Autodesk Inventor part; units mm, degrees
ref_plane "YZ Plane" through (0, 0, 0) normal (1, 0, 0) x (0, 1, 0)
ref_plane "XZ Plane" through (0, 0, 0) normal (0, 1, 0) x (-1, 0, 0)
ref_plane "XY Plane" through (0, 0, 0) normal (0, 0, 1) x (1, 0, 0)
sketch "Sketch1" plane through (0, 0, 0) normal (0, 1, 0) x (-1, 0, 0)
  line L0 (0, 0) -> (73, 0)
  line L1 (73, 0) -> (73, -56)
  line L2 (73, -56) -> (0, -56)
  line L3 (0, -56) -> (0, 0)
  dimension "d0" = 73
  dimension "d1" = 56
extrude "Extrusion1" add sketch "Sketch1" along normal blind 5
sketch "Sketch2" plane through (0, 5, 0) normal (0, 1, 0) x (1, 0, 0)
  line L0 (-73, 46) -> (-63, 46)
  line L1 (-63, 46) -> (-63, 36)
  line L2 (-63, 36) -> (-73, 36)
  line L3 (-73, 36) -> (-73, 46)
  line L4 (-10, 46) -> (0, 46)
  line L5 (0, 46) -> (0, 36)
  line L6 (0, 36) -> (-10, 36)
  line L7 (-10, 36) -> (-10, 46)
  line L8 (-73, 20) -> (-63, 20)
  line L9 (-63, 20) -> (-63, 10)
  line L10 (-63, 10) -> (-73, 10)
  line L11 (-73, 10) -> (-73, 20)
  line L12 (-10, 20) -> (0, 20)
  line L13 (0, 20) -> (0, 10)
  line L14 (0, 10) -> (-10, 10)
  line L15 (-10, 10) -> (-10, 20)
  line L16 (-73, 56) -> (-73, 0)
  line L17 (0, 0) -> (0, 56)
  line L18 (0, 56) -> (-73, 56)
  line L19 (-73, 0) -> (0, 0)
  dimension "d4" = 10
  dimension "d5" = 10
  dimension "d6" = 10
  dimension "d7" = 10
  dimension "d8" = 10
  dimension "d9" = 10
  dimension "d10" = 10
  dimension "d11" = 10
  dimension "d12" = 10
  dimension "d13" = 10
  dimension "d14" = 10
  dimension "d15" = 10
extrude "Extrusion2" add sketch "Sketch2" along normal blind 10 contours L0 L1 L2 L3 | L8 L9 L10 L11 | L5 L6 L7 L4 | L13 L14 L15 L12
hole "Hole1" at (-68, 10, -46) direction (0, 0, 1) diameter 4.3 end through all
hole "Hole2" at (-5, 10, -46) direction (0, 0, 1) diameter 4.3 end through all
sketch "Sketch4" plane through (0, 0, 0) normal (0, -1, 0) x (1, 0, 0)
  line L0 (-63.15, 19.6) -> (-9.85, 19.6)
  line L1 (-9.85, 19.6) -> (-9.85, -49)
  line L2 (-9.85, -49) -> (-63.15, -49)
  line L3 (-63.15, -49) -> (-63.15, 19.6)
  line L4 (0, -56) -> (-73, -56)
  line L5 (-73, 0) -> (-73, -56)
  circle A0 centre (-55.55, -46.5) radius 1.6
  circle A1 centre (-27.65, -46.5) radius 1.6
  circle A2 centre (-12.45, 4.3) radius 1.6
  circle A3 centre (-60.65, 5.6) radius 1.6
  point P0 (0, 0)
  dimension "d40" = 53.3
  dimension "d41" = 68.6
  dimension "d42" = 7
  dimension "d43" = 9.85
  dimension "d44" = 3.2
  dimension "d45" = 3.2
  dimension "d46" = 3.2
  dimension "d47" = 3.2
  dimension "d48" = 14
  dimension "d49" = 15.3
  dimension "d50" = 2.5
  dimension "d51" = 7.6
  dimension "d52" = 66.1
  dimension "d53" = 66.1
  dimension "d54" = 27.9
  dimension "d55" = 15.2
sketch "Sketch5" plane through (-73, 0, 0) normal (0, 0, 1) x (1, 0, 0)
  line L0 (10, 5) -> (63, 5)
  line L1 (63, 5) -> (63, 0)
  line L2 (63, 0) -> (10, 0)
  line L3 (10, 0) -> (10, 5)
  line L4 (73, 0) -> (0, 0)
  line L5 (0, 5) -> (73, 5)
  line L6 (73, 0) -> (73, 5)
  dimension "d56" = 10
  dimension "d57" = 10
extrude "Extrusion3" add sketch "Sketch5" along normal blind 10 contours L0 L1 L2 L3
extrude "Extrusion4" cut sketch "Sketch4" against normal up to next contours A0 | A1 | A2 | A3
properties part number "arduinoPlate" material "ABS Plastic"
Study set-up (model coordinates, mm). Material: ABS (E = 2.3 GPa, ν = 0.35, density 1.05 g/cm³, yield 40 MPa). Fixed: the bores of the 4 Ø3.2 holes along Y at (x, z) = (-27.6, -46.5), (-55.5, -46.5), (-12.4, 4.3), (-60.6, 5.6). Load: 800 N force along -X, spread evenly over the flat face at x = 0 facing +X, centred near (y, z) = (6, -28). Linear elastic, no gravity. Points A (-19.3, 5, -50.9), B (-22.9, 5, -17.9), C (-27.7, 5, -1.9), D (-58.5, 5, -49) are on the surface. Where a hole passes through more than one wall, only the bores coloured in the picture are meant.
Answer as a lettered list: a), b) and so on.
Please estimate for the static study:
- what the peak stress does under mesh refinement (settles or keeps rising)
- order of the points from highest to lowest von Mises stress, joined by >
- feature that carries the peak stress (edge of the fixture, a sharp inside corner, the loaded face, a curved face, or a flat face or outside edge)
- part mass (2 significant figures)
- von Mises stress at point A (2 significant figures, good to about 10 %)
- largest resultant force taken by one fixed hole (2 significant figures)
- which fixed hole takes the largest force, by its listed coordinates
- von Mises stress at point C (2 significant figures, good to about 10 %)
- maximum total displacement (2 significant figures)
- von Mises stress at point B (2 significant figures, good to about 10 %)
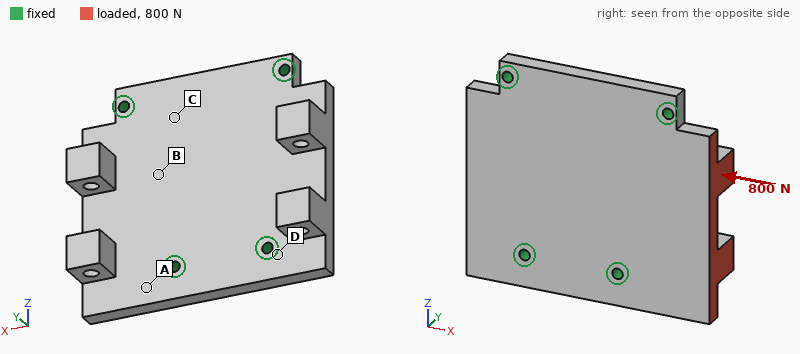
a) keeps rising
b) A > B > C > D
c) edge of the fixture
d) 28 g
e) 13 MPa
f) 370 N
g) (-27.6, -46.5)
h) 3.9 MPa
i) 0.88 mm
j) 7.8 MPa
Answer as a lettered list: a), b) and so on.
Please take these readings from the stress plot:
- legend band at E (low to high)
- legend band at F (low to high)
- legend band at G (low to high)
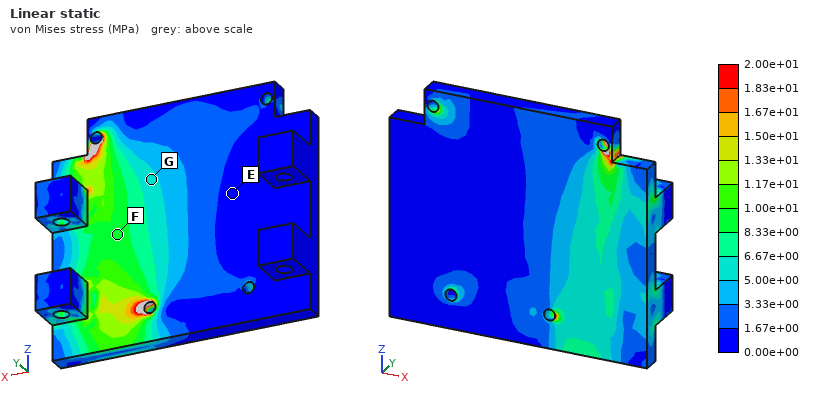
a) 0.00e+00 to 1.67e+00 MPa
b) 8.33e+00 to 1.00e+01 MPa
c) 5.00e+00 to 6.67e+00 MPa
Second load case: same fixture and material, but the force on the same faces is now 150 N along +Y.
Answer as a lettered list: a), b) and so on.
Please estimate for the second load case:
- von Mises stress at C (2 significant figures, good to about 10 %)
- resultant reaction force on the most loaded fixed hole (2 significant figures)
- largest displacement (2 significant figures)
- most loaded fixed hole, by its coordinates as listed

a) 3.3 MPa
b) 110 N
c) 1.00 mm
d) (-27.6, -46.5)
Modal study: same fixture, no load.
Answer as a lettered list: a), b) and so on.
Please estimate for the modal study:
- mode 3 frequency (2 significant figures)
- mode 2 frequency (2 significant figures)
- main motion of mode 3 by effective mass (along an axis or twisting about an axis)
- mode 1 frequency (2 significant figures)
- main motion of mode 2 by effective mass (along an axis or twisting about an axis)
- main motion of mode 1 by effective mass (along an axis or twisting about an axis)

a) 2100 Hz
b) 1700 Hz
c) along Y
d) 1200 Hz
e) along Y
f) along Y
